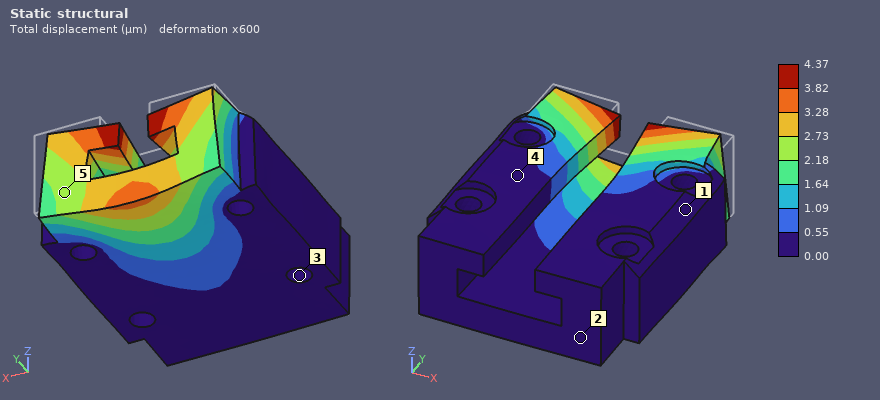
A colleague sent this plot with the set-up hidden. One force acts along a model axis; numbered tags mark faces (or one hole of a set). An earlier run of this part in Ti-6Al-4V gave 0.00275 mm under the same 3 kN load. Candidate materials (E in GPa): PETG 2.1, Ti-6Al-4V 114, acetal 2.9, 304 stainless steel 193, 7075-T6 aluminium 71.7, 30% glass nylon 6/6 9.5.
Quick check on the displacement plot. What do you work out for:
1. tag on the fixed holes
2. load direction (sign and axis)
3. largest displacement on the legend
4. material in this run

3
-Y
4.37 µm
7075-T6 aluminium
